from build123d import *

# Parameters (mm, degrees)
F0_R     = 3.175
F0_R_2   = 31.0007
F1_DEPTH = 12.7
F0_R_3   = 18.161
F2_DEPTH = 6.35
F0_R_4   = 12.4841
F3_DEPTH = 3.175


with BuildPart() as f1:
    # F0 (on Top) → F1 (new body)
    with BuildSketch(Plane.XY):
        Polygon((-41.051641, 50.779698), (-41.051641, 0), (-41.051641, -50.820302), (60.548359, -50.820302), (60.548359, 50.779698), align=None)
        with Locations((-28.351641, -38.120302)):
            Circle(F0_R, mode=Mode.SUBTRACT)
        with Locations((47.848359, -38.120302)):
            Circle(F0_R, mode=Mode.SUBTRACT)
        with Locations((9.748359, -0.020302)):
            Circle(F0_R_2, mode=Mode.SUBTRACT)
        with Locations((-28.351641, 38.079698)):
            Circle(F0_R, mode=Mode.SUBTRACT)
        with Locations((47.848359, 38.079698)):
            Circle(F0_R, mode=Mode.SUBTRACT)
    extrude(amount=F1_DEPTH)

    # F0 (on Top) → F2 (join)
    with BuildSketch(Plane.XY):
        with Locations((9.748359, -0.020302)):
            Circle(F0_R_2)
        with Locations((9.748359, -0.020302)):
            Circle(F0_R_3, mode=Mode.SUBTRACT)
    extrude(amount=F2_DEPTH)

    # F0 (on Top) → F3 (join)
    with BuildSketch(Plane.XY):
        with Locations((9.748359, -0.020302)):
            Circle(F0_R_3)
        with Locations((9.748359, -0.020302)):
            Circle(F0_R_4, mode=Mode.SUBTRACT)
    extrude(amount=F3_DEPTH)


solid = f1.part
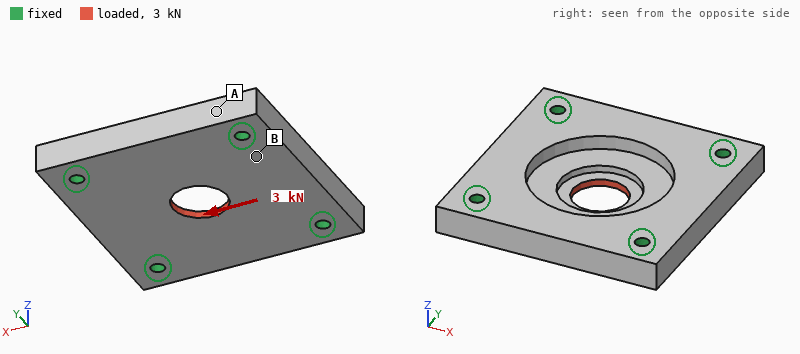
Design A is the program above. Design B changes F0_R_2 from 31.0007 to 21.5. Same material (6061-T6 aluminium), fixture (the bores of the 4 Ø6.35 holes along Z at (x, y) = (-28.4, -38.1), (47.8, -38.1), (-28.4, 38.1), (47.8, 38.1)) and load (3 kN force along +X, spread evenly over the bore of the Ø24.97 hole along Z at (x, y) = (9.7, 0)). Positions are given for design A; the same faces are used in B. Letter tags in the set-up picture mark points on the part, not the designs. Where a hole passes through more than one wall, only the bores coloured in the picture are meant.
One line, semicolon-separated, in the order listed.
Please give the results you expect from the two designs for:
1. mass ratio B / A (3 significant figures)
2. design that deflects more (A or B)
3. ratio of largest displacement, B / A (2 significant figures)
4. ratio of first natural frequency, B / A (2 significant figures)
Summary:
1.09; A; 0.81; 0.94
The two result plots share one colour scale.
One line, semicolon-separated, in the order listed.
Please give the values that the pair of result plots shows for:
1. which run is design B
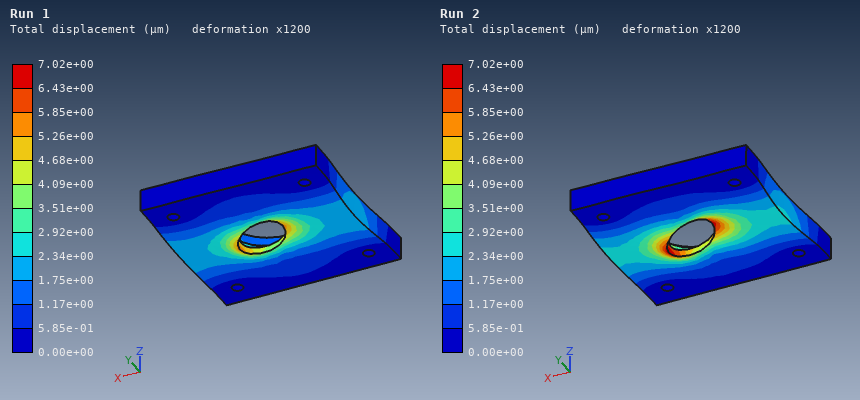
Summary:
Run 1
